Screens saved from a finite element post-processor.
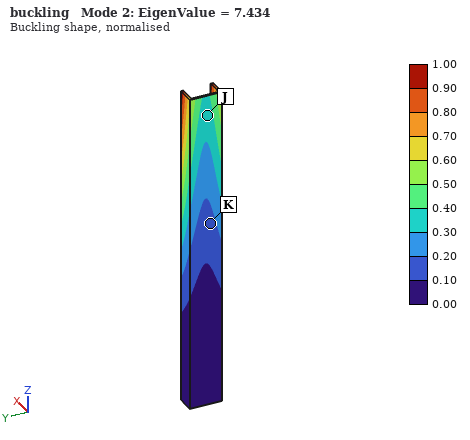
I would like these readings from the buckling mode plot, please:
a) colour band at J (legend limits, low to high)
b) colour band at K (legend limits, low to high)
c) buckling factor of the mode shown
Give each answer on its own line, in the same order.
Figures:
0.30 to 0.40
0.10 to 0.20
7.434
